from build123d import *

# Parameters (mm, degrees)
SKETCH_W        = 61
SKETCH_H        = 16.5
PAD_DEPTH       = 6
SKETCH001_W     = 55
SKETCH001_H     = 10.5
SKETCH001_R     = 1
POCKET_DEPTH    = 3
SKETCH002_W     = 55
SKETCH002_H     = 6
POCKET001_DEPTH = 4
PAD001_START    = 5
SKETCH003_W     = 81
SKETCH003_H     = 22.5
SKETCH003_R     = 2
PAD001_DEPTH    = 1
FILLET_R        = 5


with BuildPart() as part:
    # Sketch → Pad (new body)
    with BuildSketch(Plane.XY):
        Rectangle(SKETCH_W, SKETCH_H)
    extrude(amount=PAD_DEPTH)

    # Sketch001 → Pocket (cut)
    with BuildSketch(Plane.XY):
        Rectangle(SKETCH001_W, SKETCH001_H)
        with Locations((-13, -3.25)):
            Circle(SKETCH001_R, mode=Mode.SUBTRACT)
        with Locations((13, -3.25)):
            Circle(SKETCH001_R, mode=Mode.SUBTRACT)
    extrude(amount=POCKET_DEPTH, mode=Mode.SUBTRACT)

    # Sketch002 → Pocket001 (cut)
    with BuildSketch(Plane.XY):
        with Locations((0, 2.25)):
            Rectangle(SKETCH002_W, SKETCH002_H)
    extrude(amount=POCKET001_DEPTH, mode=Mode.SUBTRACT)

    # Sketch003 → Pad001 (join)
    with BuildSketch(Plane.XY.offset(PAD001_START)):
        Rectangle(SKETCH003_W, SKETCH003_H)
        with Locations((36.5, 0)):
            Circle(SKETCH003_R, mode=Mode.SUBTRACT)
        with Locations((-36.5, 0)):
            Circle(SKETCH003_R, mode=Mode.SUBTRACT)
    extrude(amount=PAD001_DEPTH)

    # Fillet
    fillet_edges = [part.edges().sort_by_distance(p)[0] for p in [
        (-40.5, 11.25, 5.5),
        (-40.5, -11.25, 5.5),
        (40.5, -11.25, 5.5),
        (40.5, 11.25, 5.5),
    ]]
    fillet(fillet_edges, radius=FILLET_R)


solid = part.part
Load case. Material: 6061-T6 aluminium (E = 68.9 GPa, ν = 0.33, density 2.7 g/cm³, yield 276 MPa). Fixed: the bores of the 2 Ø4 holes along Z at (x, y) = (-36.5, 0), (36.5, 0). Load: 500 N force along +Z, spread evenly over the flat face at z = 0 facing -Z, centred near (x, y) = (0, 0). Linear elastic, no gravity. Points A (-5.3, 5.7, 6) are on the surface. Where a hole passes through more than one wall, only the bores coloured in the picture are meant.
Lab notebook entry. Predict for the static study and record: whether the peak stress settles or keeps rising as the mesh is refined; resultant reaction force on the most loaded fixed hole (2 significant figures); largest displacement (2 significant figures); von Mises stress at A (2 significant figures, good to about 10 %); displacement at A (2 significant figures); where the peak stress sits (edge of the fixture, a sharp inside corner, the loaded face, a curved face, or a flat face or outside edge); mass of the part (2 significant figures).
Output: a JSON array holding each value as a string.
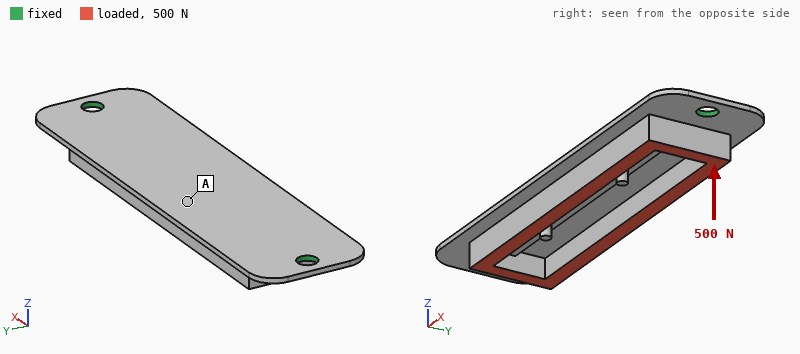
["keeps rising", "590 N", "0.15 mm", "25 MPa", "0.14 mm", "edge of the fixture", "13 g"]
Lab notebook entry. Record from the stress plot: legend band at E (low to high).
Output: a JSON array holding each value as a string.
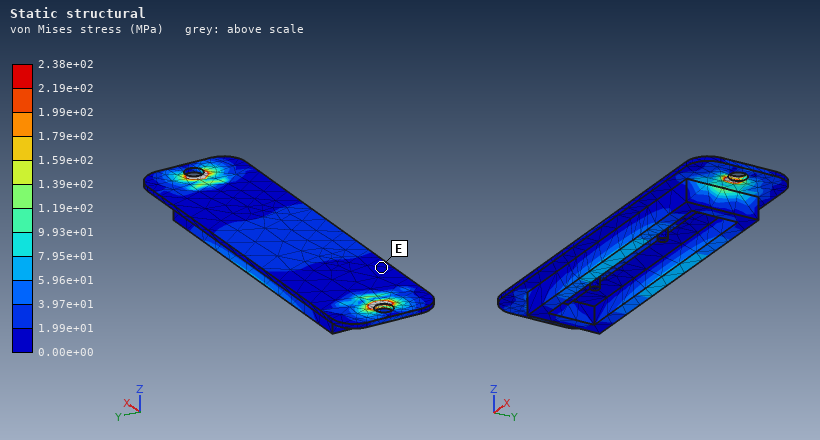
["0.00e+00 to 1.99e+01 MPa"]
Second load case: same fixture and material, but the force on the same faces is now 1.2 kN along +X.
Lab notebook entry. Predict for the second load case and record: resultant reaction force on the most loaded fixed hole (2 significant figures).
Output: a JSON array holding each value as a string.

["610 N"]
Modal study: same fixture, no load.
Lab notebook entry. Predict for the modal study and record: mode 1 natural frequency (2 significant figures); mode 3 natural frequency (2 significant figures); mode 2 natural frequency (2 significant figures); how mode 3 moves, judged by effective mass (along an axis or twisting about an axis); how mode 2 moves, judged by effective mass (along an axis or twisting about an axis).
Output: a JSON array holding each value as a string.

["2300 Hz", "6800 Hz", "2900 Hz", "twisting about Y", "along Z"]
